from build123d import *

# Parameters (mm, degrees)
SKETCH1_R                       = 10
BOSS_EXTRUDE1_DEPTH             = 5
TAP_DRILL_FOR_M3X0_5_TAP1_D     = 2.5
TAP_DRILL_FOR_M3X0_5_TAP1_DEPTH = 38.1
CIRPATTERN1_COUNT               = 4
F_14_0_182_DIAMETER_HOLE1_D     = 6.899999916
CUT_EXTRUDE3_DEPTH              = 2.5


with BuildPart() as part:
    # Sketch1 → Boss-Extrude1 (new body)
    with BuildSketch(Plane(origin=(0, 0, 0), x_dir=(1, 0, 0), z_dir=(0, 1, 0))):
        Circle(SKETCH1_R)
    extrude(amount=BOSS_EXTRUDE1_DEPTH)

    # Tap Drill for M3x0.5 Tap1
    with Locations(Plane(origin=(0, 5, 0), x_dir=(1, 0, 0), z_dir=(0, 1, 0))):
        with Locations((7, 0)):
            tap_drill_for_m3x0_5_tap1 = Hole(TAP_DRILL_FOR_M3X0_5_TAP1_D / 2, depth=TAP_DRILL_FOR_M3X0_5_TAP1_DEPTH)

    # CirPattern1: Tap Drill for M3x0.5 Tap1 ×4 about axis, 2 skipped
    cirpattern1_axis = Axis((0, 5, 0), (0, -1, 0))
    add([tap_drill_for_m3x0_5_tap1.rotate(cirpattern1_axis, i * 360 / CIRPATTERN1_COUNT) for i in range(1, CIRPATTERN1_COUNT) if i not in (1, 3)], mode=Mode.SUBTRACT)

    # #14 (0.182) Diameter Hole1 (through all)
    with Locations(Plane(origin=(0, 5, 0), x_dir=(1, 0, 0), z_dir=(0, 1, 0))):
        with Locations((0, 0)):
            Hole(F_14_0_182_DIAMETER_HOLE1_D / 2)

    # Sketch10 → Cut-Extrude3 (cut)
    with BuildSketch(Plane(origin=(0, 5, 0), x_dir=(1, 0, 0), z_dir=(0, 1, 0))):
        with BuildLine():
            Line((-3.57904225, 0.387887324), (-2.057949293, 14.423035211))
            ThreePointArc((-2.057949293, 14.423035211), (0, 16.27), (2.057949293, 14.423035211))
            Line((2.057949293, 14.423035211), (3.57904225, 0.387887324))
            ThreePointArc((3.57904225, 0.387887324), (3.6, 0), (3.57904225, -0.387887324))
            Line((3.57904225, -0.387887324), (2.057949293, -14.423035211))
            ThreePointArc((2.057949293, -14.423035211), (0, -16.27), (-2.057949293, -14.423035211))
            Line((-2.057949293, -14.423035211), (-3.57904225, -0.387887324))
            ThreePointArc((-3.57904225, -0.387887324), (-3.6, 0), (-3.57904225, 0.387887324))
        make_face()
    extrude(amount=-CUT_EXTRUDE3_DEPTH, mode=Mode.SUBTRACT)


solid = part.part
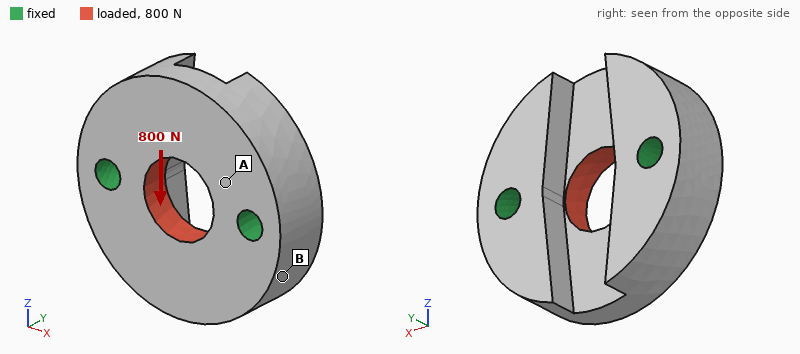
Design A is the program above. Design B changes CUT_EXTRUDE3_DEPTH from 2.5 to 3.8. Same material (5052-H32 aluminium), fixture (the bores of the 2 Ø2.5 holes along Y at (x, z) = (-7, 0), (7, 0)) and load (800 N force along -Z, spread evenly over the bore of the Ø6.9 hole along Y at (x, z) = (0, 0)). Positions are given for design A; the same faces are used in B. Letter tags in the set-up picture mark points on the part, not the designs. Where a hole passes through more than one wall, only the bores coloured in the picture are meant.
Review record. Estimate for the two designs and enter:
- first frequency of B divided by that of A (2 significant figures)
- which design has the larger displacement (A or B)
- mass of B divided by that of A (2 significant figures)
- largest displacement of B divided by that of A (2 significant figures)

1.1
B
0.90
1.6
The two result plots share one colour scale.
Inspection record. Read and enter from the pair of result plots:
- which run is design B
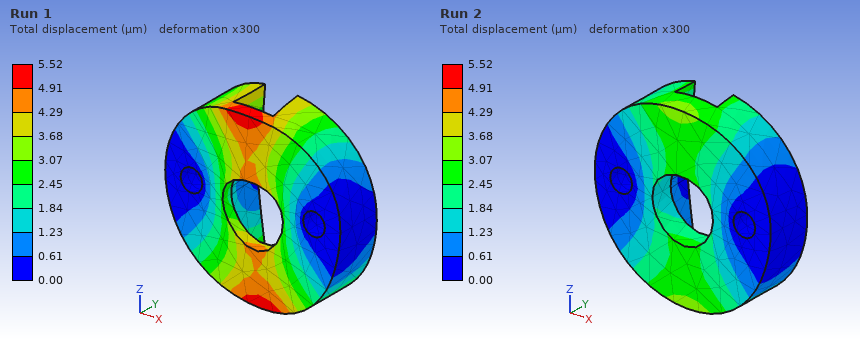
Run 1
